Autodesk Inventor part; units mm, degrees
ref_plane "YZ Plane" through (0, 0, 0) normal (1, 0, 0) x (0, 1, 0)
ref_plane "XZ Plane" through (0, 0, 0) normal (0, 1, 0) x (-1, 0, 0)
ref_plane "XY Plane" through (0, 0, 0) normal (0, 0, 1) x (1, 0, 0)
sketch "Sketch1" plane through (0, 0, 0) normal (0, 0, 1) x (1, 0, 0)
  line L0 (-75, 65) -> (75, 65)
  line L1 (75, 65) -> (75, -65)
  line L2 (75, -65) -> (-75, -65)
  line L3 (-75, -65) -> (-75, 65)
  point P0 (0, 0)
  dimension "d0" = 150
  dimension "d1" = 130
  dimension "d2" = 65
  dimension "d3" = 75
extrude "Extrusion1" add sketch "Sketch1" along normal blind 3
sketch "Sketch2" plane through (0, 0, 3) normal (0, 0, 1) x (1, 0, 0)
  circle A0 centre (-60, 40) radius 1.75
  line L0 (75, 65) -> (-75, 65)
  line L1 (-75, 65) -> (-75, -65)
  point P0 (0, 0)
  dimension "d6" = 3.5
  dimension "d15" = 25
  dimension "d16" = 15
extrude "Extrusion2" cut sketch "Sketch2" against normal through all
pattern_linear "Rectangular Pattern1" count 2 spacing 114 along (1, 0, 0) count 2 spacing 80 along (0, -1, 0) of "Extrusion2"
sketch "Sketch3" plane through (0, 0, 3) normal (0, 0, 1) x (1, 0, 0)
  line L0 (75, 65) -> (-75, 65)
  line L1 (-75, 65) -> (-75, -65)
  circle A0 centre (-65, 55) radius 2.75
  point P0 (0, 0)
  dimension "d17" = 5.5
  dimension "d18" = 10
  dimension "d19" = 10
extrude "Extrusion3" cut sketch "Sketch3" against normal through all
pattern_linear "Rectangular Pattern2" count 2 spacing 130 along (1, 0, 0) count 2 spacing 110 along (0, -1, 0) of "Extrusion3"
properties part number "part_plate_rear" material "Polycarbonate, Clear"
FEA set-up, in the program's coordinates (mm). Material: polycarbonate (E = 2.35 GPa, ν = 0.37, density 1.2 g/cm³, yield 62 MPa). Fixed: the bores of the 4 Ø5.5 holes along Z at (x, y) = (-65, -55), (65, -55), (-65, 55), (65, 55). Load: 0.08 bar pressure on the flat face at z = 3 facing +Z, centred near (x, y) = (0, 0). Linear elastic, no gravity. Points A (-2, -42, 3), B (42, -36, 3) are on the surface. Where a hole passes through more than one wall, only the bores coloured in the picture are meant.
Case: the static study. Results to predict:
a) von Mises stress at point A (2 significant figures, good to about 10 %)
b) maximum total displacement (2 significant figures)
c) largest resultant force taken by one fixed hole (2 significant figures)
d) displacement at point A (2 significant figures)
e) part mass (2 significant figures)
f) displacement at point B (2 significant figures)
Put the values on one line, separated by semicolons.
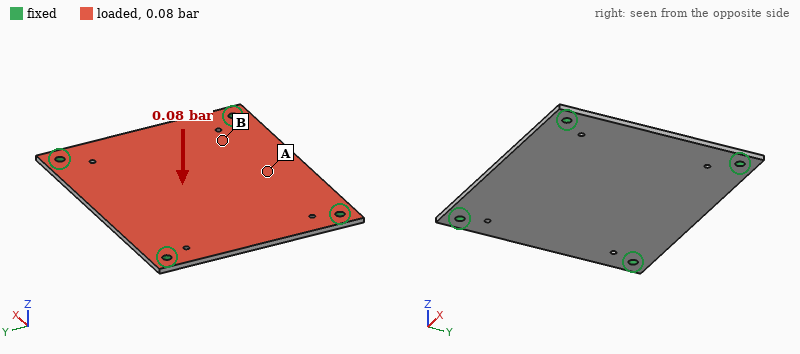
4.4 MPa; 2.2 mm; 39 N; 1.7 mm; 70 g; 0.94 mm
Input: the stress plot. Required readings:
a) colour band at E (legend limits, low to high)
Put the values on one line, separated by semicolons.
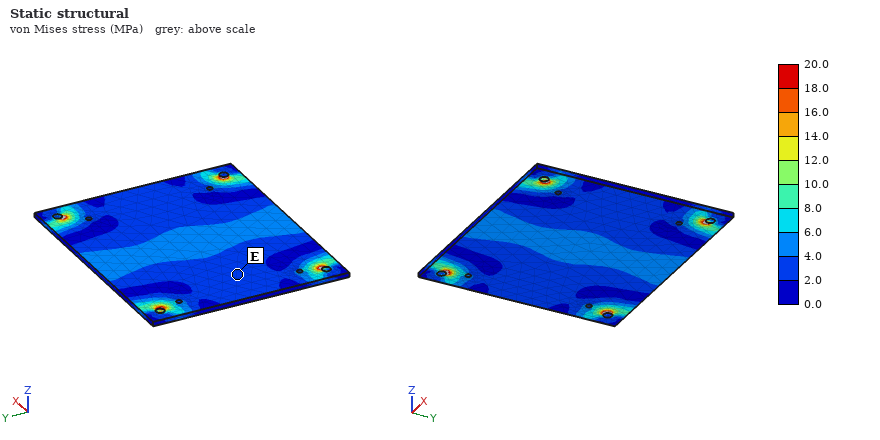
2.0 to 4.0 MPa
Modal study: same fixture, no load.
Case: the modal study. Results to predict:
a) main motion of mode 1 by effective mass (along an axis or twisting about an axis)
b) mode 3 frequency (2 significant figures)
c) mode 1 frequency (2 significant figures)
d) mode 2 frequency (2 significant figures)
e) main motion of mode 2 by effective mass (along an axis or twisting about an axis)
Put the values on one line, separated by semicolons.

along Z; 380 Hz; 190 Hz; 310 Hz; twisting about X
